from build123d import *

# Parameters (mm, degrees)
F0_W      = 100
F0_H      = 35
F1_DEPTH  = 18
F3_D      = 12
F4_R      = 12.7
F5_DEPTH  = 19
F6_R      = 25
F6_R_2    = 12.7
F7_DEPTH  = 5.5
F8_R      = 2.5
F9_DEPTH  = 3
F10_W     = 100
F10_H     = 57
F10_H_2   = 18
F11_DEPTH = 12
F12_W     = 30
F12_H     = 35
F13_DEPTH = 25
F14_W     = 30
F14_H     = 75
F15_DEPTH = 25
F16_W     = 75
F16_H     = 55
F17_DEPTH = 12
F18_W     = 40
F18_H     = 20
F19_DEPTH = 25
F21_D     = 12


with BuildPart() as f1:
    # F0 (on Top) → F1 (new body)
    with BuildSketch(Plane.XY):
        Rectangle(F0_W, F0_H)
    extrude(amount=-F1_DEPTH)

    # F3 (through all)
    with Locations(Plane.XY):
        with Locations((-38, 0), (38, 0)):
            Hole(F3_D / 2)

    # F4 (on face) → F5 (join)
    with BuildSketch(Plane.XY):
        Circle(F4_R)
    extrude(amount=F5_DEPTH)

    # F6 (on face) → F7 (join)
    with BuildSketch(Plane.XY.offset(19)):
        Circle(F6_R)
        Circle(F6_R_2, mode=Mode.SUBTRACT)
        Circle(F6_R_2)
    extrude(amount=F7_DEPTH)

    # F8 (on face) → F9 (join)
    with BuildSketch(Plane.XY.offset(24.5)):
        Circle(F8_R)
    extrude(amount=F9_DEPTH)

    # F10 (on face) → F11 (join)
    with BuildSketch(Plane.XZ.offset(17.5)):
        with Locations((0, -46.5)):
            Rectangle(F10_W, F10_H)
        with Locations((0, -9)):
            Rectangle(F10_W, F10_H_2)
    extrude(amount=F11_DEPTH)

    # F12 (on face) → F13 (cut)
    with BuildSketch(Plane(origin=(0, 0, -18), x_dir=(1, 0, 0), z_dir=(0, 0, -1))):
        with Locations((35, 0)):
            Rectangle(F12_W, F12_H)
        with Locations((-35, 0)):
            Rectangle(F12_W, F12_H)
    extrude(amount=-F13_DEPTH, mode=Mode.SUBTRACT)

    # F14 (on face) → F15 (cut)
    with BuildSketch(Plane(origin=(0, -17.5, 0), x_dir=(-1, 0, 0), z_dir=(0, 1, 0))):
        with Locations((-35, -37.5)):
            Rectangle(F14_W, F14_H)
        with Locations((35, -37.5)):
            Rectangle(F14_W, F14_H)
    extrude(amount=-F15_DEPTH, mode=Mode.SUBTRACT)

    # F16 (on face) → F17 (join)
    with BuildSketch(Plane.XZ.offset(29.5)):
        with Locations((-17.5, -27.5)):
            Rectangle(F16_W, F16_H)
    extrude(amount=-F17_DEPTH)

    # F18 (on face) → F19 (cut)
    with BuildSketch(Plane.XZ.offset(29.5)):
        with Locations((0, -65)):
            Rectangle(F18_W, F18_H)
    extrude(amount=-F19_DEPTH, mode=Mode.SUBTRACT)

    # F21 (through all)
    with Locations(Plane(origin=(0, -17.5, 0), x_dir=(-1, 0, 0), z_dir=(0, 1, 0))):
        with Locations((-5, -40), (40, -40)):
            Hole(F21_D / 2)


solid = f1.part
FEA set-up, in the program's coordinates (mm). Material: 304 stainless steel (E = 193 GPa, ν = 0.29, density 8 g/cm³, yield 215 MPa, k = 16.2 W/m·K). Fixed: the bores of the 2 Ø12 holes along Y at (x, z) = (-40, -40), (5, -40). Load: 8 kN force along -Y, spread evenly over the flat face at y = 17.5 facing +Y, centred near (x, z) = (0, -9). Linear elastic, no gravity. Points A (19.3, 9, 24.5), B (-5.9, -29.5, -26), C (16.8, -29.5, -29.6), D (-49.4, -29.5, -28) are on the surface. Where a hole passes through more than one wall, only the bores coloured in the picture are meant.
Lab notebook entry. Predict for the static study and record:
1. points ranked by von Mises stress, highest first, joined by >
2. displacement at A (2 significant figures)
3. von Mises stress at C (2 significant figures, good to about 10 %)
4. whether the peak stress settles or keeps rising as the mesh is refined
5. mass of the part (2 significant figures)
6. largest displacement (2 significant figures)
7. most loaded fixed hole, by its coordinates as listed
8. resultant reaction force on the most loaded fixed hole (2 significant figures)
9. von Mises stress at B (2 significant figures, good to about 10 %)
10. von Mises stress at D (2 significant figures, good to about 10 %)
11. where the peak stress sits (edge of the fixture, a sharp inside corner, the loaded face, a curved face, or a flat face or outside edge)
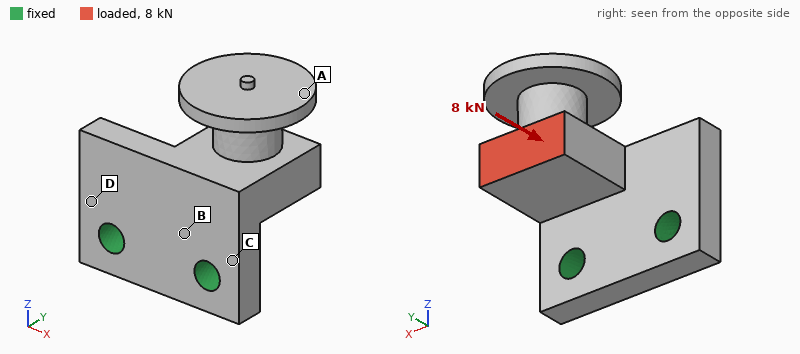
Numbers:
C > B > D > A
0.13 mm
110 MPa
keeps rising
740 g
0.14 mm
(5, -40)
6.6 kN
76 MPa
55 MPa
edge of the fixture
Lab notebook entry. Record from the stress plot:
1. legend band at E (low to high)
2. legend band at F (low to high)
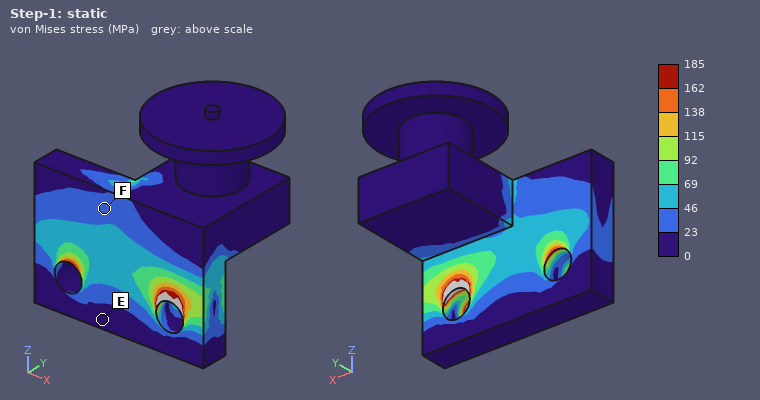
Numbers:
0 to 23 MPa
23 to 46 MPa
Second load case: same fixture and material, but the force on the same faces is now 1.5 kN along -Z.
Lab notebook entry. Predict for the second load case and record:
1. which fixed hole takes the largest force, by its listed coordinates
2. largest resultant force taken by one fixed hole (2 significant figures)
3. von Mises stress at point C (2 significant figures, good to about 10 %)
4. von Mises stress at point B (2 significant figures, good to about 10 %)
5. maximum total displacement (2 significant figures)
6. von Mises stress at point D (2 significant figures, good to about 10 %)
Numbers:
(5, -40)
1.3 kN
37 MPa
33 MPa
74 µm
21 MPa
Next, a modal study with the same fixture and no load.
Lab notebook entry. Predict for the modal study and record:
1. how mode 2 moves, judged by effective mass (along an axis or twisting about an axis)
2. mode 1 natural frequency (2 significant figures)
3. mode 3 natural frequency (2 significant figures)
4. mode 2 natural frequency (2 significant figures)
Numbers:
along X
1600 Hz
5700 Hz
3500 Hz
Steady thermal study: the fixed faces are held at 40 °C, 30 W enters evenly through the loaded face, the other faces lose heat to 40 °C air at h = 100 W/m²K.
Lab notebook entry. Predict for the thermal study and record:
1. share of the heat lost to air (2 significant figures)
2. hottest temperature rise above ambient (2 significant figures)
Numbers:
84 %
68 K
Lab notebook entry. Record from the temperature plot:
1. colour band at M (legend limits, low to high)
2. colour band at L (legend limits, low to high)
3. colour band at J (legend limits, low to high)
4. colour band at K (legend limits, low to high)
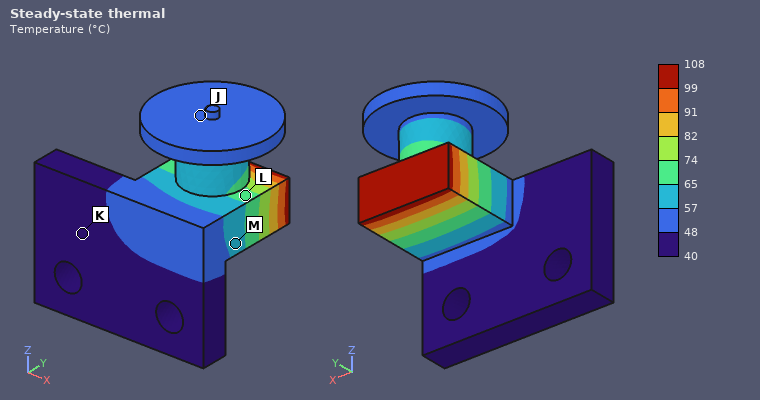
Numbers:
57 to 65 °C
65 to 74 °C
48 to 57 °C
40 to 48 °C
